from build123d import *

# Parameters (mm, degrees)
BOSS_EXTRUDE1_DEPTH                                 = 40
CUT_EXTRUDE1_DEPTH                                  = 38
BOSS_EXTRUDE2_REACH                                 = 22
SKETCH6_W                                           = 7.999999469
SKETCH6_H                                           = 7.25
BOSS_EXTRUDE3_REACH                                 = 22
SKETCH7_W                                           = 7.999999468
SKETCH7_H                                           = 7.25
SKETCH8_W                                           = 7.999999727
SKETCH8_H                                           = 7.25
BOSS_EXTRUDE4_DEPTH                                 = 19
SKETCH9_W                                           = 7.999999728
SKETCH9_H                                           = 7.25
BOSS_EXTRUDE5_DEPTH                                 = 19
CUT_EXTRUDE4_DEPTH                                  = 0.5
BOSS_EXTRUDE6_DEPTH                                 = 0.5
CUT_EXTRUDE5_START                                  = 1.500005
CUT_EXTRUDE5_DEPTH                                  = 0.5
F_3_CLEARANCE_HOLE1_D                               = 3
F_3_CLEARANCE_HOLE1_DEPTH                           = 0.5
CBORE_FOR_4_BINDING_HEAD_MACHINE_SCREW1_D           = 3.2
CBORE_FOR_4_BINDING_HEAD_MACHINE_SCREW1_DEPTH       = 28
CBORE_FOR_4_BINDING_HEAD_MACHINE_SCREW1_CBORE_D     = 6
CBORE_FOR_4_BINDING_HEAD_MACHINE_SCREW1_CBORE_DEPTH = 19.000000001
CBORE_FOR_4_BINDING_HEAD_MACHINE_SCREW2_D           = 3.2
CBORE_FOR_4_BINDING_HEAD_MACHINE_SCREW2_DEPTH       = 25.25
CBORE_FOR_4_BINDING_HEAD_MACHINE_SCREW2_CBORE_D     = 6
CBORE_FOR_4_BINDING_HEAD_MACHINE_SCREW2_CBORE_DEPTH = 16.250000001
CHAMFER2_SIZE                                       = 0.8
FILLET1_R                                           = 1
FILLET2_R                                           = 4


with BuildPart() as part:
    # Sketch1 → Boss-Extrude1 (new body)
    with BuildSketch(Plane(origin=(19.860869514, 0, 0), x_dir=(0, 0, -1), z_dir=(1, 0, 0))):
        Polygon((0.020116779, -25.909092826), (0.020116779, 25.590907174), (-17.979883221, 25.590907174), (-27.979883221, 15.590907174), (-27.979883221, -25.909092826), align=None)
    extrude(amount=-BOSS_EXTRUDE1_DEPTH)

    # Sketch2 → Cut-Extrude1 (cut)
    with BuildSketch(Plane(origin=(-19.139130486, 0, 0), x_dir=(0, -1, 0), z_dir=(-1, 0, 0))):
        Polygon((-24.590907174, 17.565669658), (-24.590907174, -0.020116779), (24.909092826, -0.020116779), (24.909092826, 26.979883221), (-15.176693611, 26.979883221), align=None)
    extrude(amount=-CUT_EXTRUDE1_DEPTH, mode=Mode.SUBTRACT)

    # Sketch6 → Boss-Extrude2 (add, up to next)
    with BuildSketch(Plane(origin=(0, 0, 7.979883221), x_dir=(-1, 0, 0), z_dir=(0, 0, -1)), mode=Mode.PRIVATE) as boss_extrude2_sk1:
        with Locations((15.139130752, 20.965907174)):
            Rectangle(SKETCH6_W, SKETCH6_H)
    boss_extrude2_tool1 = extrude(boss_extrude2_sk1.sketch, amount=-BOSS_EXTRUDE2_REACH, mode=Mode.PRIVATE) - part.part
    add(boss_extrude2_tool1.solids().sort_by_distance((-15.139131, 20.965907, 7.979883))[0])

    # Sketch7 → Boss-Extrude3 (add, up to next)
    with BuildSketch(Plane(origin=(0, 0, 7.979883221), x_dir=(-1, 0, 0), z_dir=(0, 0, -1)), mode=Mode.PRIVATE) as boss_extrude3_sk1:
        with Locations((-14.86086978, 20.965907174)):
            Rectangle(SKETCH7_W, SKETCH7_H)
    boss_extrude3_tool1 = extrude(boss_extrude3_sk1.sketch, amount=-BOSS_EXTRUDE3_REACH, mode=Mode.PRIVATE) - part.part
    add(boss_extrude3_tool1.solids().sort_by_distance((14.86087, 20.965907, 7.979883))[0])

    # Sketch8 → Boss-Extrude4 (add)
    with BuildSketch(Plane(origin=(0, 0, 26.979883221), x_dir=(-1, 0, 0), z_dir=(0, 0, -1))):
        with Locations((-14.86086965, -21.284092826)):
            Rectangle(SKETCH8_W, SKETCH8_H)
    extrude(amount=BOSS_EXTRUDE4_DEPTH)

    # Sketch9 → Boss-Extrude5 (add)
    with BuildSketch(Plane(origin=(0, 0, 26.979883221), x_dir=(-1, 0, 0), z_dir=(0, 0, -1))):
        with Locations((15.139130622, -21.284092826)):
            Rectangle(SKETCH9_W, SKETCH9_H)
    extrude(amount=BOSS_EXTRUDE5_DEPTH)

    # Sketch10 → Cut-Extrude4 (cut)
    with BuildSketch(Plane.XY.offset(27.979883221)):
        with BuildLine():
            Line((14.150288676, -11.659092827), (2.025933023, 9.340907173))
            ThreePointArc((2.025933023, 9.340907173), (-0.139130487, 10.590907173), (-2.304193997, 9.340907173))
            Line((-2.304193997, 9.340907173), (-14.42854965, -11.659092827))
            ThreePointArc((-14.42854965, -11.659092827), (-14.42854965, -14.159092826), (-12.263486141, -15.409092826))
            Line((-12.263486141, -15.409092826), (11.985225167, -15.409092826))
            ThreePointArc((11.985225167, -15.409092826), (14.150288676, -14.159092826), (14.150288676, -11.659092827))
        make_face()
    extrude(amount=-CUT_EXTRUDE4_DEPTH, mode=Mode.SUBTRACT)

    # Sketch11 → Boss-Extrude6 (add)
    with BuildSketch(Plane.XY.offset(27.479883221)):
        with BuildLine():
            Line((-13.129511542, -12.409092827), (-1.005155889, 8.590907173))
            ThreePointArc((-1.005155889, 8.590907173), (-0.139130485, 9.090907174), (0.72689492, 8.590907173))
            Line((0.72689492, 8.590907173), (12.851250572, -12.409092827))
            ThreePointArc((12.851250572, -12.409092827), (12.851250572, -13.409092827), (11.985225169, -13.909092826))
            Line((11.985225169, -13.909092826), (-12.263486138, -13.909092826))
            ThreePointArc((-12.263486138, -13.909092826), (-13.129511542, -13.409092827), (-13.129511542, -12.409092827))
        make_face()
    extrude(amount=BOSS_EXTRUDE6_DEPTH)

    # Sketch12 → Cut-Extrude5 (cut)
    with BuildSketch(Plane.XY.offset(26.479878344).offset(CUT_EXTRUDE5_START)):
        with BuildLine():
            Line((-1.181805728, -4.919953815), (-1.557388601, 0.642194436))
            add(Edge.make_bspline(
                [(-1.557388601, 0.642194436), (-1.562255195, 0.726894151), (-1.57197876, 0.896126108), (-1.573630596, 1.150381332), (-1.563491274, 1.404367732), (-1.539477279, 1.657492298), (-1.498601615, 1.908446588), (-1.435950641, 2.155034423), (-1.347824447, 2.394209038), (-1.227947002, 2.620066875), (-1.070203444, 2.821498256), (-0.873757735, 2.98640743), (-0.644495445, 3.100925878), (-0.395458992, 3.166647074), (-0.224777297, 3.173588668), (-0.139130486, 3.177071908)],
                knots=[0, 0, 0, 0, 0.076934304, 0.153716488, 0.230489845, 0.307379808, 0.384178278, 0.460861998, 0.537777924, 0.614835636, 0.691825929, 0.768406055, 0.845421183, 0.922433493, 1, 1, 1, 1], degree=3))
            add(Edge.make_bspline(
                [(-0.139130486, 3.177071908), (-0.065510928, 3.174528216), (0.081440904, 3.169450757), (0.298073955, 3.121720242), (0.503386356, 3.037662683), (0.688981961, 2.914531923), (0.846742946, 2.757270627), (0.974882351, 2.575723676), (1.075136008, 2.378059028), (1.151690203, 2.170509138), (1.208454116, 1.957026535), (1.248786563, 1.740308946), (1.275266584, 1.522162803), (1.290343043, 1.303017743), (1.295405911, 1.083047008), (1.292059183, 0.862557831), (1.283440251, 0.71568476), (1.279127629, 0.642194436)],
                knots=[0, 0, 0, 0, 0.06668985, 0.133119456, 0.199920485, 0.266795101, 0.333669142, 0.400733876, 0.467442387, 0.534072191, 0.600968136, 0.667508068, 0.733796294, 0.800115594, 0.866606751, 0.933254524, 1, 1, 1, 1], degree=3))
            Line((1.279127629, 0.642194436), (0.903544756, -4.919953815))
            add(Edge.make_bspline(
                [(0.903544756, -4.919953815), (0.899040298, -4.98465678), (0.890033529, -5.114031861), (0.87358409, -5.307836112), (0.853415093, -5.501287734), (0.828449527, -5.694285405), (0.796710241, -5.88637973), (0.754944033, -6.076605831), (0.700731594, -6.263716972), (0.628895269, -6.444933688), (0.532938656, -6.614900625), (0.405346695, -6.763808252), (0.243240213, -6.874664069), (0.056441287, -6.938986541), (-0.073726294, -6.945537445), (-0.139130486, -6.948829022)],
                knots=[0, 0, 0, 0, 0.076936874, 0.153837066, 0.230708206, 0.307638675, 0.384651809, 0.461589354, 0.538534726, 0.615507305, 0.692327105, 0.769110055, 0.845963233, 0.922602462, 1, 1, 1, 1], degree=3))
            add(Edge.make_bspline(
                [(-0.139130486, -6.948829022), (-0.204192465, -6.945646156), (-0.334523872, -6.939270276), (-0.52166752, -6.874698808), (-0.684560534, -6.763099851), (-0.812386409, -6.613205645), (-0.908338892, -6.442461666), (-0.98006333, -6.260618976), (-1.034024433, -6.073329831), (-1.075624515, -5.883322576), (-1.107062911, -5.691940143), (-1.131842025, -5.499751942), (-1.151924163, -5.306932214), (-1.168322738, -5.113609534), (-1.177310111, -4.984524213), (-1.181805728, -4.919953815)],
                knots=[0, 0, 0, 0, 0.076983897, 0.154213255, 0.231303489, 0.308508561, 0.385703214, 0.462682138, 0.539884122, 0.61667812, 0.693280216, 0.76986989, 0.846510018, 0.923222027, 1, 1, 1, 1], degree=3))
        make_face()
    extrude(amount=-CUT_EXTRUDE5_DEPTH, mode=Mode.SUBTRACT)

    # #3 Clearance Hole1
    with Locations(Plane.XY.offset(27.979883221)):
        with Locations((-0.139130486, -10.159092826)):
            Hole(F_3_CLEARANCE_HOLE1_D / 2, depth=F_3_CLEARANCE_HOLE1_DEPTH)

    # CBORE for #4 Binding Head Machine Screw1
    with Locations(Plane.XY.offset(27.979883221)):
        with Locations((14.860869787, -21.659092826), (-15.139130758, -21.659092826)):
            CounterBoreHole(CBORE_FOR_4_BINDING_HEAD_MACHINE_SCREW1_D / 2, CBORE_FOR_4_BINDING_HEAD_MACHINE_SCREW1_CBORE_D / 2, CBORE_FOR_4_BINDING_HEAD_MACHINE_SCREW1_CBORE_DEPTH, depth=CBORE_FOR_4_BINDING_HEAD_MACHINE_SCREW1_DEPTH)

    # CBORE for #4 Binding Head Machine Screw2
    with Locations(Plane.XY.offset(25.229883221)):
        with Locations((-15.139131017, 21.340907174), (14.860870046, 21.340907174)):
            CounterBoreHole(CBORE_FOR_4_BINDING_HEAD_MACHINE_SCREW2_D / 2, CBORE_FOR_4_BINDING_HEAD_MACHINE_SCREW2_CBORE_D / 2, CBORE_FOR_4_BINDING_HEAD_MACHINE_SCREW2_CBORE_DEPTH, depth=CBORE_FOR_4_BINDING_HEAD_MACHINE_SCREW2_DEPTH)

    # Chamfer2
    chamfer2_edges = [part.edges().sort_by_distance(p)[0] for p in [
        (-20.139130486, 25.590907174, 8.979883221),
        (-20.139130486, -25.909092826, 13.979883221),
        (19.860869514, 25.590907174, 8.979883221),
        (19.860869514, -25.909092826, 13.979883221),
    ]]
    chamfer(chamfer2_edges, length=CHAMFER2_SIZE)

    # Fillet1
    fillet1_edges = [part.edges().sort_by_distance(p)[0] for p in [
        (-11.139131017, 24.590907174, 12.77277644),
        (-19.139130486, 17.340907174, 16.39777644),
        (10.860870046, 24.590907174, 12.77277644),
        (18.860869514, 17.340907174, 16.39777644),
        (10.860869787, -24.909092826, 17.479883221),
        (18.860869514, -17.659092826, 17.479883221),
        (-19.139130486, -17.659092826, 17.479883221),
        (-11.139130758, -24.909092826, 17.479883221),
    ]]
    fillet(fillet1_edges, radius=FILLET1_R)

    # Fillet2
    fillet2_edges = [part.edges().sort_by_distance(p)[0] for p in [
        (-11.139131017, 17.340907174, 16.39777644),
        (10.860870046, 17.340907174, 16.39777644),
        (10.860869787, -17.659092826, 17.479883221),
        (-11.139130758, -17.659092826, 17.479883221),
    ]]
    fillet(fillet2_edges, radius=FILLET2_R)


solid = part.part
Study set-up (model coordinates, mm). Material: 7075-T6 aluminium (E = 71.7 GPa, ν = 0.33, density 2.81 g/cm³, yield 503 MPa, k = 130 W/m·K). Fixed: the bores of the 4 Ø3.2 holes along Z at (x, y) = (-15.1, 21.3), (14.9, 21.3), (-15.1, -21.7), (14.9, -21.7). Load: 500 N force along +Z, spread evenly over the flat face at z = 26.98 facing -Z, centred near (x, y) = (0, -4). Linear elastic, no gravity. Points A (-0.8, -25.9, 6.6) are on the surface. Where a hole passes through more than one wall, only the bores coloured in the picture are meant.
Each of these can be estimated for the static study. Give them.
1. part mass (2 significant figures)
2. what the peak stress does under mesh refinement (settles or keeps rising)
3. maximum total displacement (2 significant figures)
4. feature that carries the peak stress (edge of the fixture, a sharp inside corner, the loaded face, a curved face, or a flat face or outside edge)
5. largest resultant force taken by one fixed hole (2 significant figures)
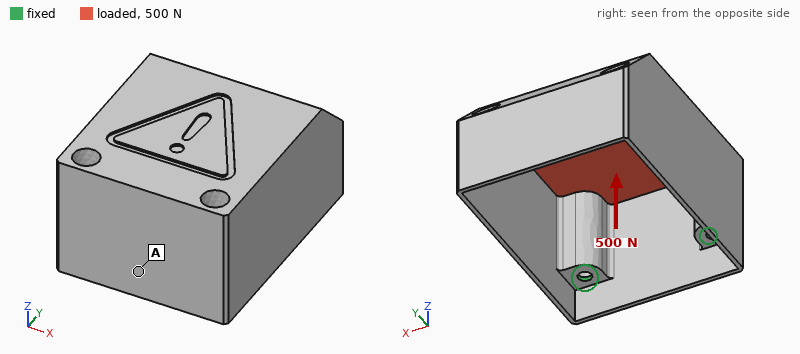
23 g
keeps rising
0.27 mm
a sharp inside corner
150 N
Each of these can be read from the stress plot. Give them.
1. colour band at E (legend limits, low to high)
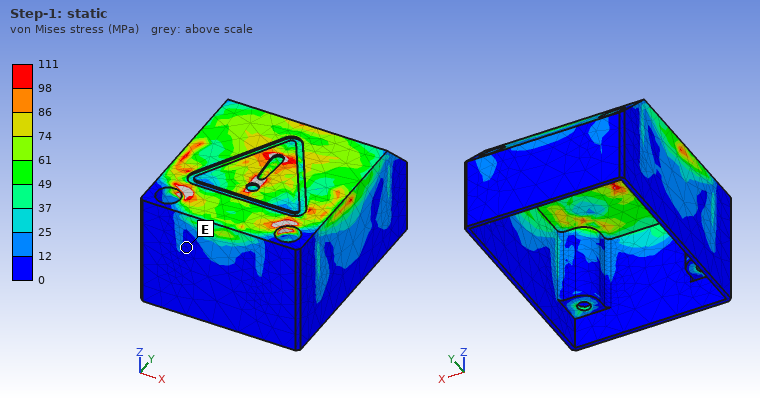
0 to 12 MPa
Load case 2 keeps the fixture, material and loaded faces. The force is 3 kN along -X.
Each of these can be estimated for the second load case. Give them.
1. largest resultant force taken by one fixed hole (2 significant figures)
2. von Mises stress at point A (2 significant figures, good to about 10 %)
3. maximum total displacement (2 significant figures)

1.2 kN
32 MPa
90 µm
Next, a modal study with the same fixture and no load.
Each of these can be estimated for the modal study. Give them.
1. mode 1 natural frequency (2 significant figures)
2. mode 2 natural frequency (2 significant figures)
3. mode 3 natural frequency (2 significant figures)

4000 Hz
4000 Hz
4700 Hz
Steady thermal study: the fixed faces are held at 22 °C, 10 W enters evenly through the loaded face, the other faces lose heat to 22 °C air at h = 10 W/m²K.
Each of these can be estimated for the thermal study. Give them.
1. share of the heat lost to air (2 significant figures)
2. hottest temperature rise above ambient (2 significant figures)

8.2 %
17 K
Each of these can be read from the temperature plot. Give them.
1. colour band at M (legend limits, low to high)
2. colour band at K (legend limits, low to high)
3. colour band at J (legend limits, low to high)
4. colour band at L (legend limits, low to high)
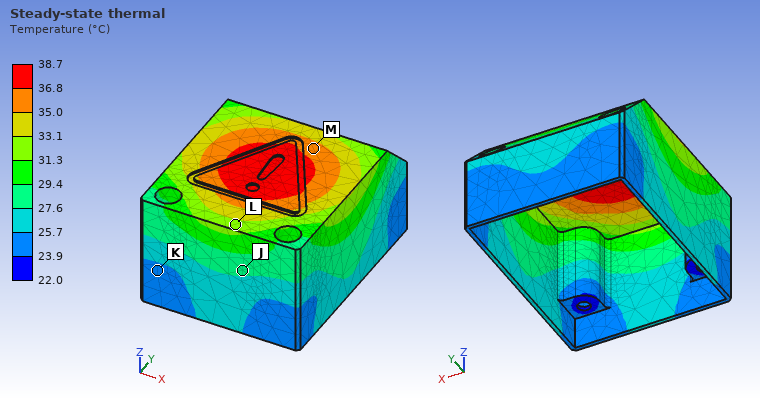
35.0 to 36.8 °C
23.9 to 25.7 °C
27.6 to 29.4 °C
31.3 to 33.1 °C
